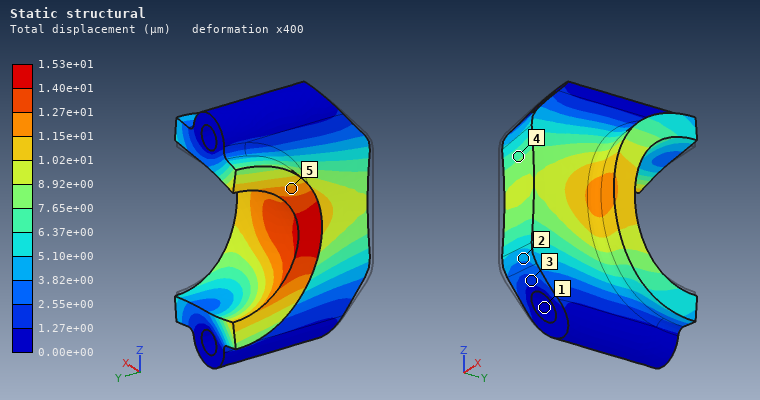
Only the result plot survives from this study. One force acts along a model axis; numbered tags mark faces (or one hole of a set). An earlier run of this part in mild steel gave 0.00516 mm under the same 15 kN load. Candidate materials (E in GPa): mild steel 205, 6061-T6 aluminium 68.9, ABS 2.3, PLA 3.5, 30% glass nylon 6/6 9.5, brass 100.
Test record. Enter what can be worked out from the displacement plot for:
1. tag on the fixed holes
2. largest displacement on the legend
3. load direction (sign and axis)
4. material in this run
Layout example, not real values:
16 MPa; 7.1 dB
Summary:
1; 1.53e+01 µm; +X; 6061-T6 aluminium
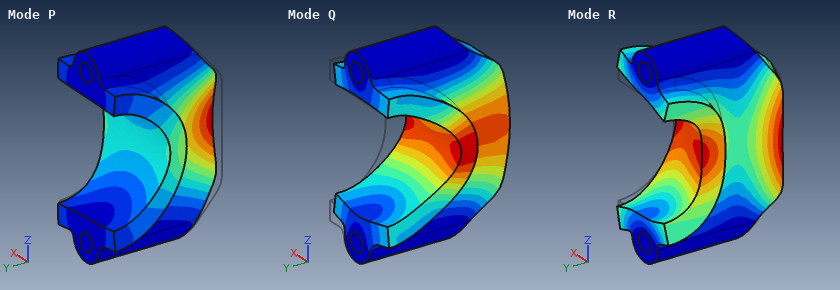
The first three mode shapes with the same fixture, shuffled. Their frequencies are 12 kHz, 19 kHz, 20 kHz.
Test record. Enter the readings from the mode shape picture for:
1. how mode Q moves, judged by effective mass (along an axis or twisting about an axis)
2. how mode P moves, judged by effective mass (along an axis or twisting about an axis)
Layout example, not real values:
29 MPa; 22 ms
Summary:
along Y; along X
